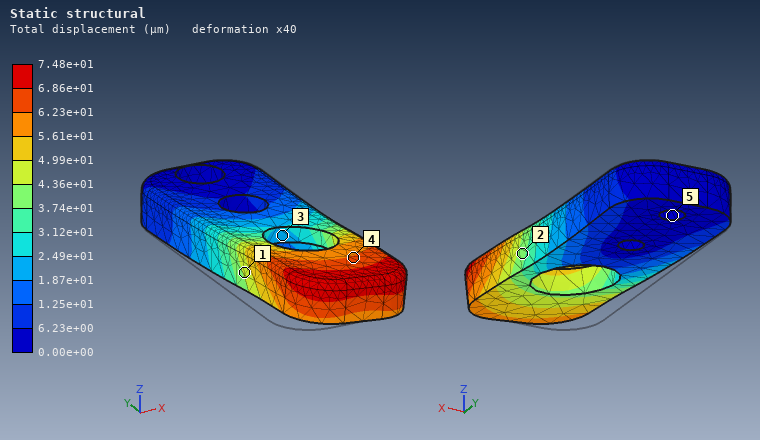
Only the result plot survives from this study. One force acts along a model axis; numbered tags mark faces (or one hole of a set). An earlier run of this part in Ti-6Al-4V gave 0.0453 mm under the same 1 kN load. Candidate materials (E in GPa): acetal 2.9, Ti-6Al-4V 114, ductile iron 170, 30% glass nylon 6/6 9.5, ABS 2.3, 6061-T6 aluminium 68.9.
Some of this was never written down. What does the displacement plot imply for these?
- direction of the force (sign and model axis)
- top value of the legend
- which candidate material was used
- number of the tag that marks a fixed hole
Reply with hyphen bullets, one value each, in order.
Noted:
- +X
- 7.48e+01 µm
- 6061-T6 aluminium
- 5
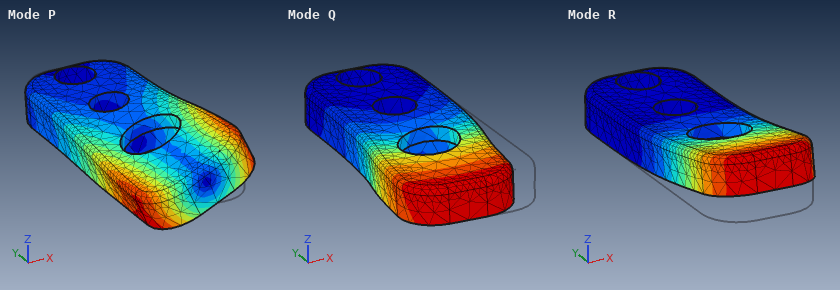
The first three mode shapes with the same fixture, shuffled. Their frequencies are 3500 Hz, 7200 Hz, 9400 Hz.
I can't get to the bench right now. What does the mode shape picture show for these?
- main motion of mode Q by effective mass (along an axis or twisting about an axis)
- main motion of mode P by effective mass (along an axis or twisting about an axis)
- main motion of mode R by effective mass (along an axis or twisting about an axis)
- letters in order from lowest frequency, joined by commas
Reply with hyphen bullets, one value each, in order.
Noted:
- along X
- twisting about Y
- along Z
- R, Q, P
